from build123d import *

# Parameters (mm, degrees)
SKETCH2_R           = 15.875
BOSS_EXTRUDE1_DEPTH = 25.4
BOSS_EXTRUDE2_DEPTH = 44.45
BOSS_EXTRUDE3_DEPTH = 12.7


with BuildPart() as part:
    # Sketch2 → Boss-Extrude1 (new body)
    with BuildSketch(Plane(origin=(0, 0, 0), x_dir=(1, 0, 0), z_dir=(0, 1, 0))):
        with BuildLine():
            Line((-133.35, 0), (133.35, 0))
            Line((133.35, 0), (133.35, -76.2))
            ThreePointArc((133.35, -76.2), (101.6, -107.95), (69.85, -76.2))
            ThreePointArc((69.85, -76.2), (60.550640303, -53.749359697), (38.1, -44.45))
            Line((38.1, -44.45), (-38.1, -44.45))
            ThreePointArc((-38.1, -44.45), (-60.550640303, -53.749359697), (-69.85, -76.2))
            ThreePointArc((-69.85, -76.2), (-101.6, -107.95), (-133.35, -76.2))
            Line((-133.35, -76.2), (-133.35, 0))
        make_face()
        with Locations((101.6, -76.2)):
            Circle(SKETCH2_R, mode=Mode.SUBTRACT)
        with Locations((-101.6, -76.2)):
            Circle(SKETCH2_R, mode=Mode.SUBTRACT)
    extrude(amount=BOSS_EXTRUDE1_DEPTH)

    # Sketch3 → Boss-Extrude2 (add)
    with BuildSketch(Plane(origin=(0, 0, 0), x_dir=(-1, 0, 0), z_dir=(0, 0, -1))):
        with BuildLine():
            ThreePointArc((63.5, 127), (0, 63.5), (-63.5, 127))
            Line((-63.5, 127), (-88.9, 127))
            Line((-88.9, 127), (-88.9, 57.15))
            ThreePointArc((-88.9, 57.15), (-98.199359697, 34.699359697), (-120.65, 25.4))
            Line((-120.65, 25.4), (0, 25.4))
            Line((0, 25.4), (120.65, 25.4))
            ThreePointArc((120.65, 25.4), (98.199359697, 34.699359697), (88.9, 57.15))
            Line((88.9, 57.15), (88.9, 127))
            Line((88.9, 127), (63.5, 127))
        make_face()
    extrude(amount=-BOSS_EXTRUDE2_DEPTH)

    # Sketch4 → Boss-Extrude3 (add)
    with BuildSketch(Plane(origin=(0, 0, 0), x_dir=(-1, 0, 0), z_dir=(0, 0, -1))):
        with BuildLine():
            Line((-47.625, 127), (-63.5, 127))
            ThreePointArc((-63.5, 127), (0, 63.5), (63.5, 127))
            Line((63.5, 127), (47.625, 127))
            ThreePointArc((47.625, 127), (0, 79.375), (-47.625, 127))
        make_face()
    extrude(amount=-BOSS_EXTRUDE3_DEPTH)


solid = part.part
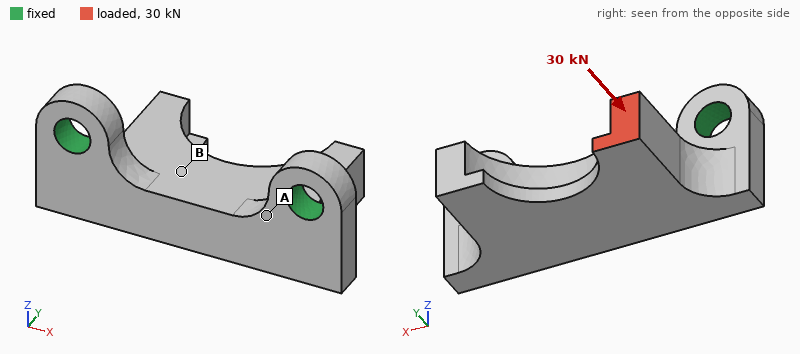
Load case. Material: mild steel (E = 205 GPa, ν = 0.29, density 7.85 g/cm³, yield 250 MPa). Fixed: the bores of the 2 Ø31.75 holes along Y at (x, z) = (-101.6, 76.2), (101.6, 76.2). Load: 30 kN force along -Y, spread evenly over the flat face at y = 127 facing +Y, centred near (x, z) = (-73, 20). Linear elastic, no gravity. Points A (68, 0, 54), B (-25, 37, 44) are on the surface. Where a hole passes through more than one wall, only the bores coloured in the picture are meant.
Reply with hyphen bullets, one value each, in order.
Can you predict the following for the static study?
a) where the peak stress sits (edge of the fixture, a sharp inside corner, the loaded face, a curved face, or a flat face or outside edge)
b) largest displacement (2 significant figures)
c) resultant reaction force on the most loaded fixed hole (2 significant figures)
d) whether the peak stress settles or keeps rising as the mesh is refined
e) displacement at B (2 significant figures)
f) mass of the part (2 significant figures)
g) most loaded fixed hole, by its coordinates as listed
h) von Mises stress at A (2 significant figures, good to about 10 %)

- edge of the fixture
- 0.14 mm
- 26 kN
- keeps rising
- 0.030 mm
- 8.1 kg
- (-101.6, 76.2)
- 42 MPa
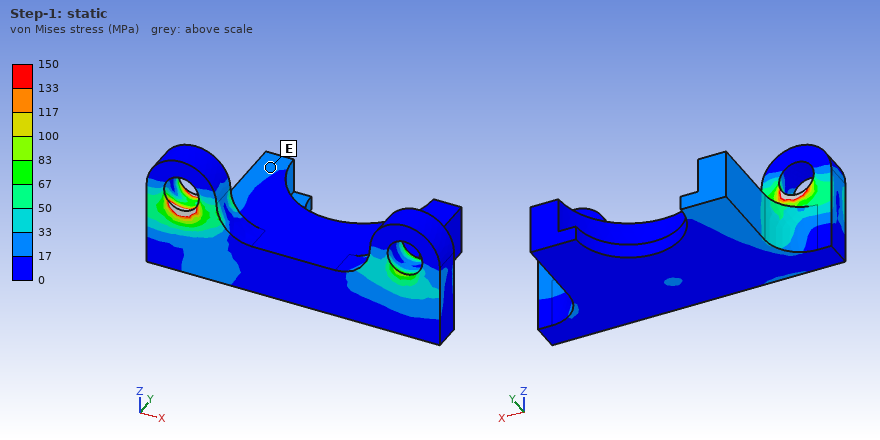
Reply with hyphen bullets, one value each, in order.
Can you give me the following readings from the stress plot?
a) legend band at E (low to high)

- 17 to 33 MPa
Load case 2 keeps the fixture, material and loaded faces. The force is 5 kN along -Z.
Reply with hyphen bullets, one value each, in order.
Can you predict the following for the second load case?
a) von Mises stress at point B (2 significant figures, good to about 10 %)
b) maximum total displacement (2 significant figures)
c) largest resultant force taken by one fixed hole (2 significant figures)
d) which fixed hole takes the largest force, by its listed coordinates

- 13 MPa
- 0.11 mm
- 4.6 kN
- (-101.6, 76.2)
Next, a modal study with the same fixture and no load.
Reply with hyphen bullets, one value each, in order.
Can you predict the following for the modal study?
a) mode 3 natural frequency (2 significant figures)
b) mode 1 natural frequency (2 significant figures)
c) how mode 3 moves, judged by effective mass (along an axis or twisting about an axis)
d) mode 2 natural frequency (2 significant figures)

- 3200 Hz
- 1000 Hz
- along Y
- 2300 Hz
